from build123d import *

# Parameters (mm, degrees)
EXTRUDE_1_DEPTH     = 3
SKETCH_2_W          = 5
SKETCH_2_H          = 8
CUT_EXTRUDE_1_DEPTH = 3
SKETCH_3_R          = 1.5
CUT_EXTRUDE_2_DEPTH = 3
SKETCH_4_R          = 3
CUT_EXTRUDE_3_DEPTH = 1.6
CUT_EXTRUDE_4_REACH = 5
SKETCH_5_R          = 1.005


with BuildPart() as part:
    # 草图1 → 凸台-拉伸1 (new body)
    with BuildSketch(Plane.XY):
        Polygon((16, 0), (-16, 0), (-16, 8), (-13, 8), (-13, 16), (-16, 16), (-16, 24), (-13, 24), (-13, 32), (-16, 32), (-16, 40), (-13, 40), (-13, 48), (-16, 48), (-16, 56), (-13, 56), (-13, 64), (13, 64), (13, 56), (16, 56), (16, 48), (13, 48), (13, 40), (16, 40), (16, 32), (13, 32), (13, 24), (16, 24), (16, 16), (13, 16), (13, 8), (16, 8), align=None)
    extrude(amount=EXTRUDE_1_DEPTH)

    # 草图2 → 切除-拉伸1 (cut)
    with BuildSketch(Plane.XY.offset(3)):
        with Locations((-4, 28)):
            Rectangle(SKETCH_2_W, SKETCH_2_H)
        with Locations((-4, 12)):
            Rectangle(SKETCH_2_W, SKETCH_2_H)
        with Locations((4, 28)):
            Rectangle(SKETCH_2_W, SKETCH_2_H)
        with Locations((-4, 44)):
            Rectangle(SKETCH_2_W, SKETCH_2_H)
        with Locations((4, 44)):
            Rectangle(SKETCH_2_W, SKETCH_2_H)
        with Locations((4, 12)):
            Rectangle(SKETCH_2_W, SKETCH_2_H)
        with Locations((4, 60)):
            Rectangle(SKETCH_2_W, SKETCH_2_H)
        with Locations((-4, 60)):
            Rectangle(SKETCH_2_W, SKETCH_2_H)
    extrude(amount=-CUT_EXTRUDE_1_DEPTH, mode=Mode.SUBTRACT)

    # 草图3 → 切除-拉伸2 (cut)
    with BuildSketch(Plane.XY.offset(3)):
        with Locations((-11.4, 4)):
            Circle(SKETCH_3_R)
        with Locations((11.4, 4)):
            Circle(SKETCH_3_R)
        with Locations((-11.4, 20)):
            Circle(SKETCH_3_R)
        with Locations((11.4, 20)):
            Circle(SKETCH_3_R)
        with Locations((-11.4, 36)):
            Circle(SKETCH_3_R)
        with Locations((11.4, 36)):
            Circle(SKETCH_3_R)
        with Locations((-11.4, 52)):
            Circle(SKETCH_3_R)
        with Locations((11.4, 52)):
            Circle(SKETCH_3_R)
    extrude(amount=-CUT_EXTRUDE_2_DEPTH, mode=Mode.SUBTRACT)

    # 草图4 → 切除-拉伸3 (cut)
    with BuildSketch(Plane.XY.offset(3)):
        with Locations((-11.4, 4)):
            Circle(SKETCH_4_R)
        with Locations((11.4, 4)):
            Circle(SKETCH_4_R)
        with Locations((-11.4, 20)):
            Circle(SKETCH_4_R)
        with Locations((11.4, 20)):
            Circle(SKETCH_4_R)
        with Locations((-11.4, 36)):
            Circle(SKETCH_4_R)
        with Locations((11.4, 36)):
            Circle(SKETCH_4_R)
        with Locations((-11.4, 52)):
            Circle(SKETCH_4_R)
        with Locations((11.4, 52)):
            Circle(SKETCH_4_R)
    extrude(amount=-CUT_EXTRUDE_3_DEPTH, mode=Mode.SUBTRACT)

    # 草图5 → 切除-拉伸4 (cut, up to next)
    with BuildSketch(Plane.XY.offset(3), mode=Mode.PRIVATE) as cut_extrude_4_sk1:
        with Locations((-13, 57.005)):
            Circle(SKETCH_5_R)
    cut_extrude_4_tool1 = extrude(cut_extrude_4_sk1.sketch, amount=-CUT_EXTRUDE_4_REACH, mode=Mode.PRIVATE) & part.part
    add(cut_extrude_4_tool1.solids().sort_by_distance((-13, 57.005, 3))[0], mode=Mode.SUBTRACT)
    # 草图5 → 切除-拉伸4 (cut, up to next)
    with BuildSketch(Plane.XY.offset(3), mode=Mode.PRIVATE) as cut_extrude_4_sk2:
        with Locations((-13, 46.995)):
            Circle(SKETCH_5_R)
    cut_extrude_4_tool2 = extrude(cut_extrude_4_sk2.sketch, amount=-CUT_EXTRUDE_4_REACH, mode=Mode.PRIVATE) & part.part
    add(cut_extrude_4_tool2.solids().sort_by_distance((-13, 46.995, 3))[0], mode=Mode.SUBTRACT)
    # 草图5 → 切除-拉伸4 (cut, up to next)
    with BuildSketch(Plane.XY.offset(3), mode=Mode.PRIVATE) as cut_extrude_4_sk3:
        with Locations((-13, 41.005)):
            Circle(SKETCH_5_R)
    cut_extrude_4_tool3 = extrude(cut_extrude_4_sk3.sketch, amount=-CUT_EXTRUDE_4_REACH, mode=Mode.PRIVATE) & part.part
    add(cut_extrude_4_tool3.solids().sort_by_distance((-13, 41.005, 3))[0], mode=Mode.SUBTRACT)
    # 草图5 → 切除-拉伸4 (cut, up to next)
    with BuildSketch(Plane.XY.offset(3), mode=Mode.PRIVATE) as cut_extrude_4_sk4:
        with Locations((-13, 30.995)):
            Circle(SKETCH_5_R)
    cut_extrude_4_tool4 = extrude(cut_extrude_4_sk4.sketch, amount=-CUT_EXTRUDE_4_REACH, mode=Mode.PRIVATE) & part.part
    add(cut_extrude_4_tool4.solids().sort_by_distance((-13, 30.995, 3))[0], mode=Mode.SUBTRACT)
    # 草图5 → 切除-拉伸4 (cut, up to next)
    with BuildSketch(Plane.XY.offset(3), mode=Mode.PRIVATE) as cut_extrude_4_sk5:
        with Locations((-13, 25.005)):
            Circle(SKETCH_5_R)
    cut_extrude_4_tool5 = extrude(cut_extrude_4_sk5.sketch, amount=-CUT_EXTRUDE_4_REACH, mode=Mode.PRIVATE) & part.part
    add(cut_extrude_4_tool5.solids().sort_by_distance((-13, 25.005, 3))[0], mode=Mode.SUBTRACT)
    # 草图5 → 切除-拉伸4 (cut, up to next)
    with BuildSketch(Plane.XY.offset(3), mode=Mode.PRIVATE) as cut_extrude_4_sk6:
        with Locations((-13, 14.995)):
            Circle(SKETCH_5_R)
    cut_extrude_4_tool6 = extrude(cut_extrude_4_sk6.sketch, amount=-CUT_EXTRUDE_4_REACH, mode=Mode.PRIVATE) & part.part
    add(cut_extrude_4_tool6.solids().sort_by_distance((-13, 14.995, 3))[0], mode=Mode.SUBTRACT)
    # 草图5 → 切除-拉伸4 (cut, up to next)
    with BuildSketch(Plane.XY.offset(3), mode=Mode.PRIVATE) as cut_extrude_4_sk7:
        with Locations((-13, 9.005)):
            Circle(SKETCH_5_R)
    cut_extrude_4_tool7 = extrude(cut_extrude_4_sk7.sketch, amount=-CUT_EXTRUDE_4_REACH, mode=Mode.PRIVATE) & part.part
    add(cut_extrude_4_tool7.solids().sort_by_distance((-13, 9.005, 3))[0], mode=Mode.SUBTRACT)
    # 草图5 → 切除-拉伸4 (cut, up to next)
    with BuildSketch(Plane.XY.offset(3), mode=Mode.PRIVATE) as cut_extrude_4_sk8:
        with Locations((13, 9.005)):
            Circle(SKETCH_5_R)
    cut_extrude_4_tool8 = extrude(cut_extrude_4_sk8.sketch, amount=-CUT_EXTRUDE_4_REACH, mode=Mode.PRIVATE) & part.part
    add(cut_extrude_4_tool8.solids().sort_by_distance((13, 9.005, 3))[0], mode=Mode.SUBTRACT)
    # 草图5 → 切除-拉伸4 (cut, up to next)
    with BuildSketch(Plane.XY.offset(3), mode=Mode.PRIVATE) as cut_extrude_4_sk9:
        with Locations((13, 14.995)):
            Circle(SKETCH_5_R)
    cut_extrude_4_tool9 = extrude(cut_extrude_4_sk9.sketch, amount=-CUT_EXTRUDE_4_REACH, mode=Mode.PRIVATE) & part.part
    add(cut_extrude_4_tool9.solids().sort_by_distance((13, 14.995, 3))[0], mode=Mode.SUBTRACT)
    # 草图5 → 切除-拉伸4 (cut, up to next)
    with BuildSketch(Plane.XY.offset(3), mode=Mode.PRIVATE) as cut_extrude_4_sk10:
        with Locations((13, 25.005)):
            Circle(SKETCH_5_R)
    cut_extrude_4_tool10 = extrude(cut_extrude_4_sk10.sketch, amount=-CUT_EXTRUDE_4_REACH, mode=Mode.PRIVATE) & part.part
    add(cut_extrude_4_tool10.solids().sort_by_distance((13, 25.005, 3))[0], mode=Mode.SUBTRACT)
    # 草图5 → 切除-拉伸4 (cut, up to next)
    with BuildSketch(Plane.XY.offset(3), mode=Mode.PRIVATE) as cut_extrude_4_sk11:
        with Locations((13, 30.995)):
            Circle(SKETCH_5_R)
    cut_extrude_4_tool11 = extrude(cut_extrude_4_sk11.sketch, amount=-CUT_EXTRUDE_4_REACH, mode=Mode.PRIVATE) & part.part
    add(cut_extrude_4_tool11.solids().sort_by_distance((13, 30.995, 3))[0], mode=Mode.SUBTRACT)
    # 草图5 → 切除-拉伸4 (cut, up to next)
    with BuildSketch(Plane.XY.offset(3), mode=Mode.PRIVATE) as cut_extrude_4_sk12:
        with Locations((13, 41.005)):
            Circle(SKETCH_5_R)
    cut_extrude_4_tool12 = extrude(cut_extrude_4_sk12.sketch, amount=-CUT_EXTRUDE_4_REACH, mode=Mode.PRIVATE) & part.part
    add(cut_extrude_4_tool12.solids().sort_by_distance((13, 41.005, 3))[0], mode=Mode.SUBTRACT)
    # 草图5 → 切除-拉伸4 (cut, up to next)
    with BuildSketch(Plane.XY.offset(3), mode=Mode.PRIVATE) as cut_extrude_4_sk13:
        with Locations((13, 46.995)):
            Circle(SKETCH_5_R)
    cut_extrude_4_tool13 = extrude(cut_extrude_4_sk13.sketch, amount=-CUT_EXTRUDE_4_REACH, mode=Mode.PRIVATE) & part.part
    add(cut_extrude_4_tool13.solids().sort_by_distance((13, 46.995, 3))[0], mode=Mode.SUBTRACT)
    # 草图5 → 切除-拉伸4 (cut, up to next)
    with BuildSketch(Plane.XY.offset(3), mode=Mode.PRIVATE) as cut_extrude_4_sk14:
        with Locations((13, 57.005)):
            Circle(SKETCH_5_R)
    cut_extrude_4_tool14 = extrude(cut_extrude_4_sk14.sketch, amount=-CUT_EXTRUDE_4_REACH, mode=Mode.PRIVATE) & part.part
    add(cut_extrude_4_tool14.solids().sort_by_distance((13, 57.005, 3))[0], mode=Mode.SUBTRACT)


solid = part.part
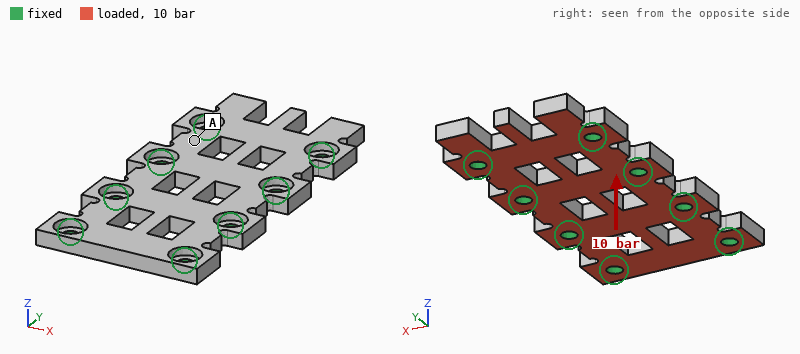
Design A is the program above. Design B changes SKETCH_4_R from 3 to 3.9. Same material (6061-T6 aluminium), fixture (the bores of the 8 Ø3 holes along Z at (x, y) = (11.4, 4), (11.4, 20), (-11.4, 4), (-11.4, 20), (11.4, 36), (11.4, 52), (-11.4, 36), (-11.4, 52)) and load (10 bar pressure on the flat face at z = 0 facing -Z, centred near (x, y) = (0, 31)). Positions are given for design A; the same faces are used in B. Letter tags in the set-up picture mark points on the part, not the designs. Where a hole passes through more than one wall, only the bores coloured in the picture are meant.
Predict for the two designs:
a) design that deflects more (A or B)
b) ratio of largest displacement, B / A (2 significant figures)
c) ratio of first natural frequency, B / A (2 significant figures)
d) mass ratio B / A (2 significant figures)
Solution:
B
1.2
0.89
0.94
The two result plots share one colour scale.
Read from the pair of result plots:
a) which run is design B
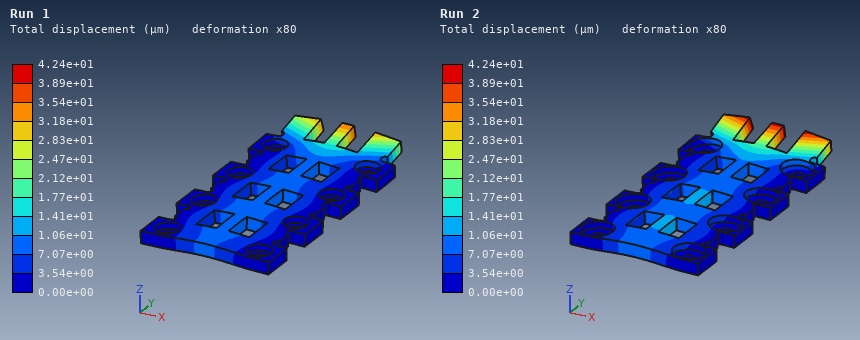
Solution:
Run 2
